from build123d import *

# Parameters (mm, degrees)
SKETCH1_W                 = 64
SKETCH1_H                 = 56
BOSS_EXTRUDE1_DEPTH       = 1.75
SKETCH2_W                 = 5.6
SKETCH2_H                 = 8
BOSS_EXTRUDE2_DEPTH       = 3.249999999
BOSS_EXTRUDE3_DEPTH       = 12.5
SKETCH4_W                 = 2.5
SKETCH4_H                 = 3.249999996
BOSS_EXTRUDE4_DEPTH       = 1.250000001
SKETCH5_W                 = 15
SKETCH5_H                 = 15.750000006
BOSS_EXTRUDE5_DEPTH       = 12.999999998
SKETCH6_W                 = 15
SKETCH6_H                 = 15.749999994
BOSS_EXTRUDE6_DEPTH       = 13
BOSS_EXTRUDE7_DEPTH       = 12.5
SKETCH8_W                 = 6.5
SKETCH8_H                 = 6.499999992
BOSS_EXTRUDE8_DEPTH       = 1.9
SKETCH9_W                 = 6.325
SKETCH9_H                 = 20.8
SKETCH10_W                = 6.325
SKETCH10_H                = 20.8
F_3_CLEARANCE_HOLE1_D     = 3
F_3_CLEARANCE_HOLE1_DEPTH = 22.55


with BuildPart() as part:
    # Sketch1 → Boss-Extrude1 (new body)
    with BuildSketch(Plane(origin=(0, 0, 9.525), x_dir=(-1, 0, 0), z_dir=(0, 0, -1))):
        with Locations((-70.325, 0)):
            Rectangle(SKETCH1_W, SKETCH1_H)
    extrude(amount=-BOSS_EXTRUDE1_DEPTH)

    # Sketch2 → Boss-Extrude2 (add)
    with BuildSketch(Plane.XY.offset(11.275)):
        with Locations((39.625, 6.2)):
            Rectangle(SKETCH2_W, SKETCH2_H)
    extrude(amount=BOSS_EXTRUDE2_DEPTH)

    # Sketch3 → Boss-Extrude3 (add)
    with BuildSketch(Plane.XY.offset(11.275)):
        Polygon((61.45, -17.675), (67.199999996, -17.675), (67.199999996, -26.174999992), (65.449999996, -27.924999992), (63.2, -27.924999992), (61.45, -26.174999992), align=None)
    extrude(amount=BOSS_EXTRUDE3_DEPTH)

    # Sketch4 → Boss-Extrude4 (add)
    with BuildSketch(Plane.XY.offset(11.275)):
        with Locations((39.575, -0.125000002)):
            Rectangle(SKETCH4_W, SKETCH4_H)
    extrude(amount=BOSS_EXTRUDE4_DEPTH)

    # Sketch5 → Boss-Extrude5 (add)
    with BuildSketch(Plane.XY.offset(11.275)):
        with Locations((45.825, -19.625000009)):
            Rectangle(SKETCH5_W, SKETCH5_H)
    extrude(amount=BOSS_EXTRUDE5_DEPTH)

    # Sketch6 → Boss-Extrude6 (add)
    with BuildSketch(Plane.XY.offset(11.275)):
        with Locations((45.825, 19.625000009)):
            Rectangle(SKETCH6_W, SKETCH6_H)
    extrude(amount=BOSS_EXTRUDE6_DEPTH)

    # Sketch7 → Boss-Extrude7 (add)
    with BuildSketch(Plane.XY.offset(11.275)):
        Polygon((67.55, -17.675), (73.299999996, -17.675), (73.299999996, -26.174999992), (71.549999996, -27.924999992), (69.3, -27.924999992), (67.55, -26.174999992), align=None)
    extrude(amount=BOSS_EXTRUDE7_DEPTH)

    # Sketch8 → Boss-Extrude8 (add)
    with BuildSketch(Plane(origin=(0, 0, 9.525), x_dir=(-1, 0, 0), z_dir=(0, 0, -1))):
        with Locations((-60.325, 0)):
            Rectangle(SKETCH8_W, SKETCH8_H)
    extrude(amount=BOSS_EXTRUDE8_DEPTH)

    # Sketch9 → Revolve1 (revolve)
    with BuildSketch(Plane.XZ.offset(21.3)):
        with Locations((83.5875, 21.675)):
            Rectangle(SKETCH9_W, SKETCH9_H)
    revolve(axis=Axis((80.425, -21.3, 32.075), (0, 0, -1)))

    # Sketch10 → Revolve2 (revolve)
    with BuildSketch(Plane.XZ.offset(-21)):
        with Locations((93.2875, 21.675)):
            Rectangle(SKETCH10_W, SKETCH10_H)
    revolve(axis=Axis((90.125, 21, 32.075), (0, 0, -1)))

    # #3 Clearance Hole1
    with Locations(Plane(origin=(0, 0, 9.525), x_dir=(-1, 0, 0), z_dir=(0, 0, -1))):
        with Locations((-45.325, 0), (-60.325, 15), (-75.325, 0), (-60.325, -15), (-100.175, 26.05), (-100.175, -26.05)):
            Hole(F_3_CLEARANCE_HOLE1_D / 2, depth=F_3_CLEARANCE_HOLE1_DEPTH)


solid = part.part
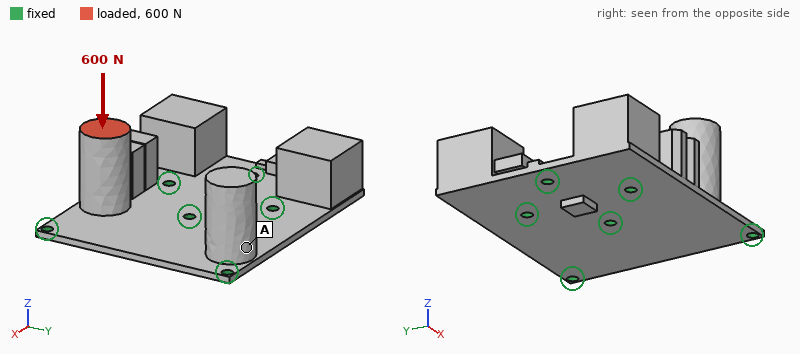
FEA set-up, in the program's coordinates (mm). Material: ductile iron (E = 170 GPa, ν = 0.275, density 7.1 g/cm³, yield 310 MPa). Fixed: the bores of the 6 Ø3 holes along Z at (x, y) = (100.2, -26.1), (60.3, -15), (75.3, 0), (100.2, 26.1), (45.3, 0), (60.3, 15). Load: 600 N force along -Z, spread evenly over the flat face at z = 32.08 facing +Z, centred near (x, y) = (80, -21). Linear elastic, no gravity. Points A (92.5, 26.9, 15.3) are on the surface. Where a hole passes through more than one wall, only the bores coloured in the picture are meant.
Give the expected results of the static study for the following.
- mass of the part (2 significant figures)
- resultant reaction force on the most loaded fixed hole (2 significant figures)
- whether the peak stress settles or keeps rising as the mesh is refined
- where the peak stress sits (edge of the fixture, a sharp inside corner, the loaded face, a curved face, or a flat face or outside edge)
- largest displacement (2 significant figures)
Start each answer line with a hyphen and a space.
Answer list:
- 140 g
- 310 N
- keeps rising
- edge of the fixture
- 0.12 mm
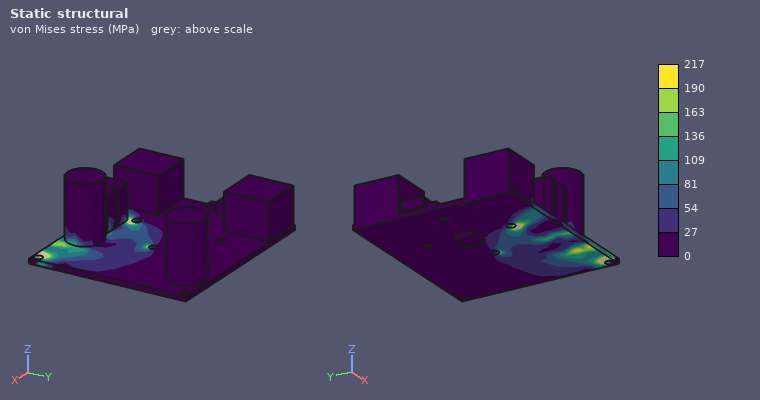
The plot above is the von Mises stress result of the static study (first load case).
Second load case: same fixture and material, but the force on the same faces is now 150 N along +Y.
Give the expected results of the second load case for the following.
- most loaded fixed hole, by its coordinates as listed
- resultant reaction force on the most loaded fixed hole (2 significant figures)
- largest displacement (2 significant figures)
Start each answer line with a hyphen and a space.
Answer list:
- (75.3, 0)
- 140 N
- 100 µm
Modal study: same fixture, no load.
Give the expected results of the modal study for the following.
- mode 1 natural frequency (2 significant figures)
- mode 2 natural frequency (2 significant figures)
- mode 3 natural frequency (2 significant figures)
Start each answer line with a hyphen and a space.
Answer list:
- 1600 Hz
- 1600 Hz
- 2000 Hz
